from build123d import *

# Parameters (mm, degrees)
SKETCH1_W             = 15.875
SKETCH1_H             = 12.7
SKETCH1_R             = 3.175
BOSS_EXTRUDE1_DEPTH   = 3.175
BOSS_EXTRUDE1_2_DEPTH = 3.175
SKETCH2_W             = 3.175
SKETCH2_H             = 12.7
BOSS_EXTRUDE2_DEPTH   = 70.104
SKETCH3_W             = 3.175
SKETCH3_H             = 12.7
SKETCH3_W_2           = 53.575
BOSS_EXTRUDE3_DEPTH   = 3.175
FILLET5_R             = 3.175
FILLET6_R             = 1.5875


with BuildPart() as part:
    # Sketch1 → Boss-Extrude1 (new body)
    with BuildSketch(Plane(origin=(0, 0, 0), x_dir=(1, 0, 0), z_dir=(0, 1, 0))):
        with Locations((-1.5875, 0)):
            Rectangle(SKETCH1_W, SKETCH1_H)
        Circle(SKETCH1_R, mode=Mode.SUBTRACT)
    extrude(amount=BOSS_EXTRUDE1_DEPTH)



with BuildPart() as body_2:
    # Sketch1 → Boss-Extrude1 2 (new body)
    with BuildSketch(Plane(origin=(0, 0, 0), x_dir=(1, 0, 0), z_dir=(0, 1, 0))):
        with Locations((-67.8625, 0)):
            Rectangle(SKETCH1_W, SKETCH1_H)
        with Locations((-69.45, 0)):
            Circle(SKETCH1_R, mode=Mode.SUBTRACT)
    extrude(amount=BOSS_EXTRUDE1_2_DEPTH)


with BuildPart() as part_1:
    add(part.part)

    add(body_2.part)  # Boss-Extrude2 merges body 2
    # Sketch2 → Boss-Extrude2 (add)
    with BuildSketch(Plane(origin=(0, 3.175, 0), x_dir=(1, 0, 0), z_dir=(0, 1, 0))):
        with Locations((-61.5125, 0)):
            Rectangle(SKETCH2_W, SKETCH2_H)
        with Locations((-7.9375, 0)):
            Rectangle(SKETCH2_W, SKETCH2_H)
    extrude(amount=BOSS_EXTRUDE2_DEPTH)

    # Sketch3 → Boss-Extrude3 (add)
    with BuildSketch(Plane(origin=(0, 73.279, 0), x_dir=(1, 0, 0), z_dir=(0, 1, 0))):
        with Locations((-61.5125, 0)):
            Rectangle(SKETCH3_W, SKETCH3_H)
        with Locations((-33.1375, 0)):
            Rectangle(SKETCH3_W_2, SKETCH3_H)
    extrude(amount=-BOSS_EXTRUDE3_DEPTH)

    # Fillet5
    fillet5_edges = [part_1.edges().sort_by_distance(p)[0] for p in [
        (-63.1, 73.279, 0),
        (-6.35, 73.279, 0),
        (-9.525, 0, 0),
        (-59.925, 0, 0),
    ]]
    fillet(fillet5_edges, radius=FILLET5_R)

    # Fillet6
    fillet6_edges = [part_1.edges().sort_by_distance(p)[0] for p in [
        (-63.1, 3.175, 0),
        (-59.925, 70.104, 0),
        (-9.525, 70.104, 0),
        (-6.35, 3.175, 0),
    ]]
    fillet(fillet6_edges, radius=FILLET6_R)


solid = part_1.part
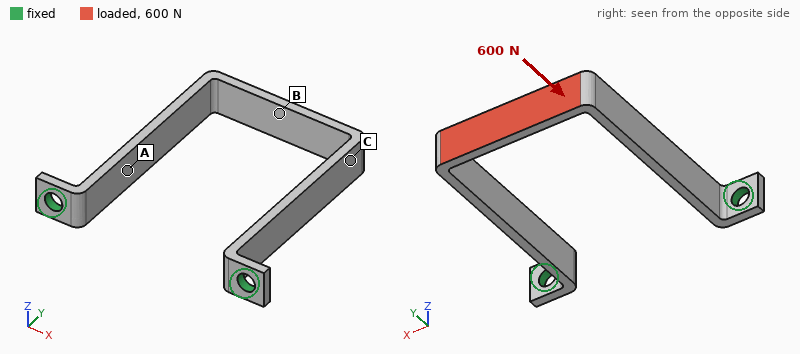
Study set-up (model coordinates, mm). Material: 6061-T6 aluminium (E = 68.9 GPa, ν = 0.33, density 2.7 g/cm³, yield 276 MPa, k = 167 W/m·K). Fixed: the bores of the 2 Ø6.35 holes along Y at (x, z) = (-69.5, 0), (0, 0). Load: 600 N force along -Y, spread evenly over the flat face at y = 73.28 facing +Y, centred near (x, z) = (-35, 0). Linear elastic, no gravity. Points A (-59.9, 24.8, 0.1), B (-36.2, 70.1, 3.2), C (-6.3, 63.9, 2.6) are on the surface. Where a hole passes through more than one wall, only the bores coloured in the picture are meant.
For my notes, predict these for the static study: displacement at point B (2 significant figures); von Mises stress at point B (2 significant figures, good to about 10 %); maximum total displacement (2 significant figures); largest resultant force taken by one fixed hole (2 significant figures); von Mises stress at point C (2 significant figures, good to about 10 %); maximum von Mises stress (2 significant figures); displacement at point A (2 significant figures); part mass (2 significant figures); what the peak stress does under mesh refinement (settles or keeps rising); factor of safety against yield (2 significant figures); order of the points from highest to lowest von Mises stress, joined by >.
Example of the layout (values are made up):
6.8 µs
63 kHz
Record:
0.27 mm
110 MPa
0.28 mm
300 N
61 MPa
120 MPa
0.061 mm
23 g
settles
2.4
B > C > A
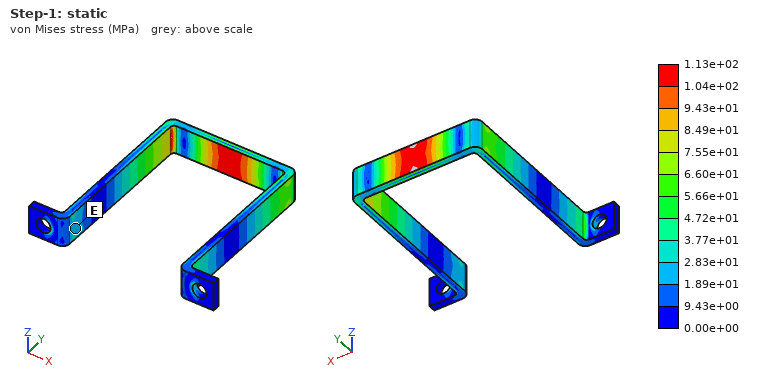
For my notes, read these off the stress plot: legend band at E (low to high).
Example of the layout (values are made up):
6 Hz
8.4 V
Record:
1.89e+01 to 2.83e+01 MPa
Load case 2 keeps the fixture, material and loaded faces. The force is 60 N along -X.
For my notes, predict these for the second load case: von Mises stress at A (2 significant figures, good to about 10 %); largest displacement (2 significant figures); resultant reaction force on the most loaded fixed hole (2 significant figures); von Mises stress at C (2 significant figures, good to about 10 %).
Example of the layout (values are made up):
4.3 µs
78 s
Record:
18 MPa
0.51 mm
49 N
34 MPa
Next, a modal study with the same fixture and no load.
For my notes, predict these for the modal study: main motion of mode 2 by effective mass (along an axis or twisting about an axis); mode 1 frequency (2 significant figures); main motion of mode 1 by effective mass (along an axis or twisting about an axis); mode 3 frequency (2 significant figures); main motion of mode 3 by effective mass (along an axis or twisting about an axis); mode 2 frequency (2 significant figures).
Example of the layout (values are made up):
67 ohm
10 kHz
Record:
along Z
520 Hz
along X
1300 Hz
twisting about Y
790 Hz
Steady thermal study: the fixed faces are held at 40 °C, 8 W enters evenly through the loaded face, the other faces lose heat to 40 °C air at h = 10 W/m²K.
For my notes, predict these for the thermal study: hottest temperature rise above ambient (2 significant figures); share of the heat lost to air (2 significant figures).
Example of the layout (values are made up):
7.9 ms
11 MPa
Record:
45 K
16 %
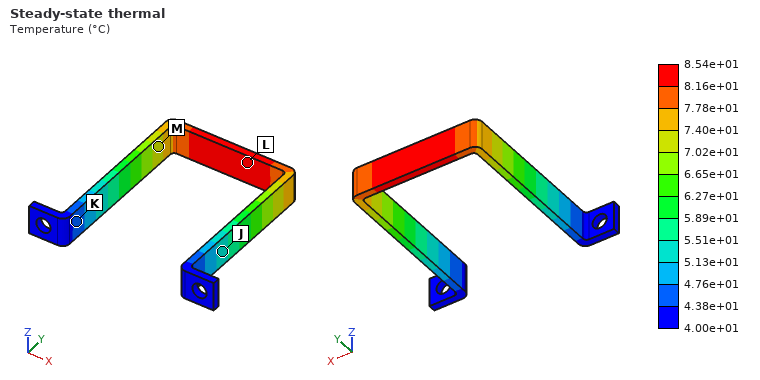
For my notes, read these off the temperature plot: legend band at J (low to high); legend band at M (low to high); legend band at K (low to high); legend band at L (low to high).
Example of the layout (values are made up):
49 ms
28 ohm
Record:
5.13e+01 to 5.51e+01 °C
7.02e+01 to 7.40e+01 °C
4.38e+01 to 4.76e+01 °C
8.16e+01 to 8.54e+01 °C
